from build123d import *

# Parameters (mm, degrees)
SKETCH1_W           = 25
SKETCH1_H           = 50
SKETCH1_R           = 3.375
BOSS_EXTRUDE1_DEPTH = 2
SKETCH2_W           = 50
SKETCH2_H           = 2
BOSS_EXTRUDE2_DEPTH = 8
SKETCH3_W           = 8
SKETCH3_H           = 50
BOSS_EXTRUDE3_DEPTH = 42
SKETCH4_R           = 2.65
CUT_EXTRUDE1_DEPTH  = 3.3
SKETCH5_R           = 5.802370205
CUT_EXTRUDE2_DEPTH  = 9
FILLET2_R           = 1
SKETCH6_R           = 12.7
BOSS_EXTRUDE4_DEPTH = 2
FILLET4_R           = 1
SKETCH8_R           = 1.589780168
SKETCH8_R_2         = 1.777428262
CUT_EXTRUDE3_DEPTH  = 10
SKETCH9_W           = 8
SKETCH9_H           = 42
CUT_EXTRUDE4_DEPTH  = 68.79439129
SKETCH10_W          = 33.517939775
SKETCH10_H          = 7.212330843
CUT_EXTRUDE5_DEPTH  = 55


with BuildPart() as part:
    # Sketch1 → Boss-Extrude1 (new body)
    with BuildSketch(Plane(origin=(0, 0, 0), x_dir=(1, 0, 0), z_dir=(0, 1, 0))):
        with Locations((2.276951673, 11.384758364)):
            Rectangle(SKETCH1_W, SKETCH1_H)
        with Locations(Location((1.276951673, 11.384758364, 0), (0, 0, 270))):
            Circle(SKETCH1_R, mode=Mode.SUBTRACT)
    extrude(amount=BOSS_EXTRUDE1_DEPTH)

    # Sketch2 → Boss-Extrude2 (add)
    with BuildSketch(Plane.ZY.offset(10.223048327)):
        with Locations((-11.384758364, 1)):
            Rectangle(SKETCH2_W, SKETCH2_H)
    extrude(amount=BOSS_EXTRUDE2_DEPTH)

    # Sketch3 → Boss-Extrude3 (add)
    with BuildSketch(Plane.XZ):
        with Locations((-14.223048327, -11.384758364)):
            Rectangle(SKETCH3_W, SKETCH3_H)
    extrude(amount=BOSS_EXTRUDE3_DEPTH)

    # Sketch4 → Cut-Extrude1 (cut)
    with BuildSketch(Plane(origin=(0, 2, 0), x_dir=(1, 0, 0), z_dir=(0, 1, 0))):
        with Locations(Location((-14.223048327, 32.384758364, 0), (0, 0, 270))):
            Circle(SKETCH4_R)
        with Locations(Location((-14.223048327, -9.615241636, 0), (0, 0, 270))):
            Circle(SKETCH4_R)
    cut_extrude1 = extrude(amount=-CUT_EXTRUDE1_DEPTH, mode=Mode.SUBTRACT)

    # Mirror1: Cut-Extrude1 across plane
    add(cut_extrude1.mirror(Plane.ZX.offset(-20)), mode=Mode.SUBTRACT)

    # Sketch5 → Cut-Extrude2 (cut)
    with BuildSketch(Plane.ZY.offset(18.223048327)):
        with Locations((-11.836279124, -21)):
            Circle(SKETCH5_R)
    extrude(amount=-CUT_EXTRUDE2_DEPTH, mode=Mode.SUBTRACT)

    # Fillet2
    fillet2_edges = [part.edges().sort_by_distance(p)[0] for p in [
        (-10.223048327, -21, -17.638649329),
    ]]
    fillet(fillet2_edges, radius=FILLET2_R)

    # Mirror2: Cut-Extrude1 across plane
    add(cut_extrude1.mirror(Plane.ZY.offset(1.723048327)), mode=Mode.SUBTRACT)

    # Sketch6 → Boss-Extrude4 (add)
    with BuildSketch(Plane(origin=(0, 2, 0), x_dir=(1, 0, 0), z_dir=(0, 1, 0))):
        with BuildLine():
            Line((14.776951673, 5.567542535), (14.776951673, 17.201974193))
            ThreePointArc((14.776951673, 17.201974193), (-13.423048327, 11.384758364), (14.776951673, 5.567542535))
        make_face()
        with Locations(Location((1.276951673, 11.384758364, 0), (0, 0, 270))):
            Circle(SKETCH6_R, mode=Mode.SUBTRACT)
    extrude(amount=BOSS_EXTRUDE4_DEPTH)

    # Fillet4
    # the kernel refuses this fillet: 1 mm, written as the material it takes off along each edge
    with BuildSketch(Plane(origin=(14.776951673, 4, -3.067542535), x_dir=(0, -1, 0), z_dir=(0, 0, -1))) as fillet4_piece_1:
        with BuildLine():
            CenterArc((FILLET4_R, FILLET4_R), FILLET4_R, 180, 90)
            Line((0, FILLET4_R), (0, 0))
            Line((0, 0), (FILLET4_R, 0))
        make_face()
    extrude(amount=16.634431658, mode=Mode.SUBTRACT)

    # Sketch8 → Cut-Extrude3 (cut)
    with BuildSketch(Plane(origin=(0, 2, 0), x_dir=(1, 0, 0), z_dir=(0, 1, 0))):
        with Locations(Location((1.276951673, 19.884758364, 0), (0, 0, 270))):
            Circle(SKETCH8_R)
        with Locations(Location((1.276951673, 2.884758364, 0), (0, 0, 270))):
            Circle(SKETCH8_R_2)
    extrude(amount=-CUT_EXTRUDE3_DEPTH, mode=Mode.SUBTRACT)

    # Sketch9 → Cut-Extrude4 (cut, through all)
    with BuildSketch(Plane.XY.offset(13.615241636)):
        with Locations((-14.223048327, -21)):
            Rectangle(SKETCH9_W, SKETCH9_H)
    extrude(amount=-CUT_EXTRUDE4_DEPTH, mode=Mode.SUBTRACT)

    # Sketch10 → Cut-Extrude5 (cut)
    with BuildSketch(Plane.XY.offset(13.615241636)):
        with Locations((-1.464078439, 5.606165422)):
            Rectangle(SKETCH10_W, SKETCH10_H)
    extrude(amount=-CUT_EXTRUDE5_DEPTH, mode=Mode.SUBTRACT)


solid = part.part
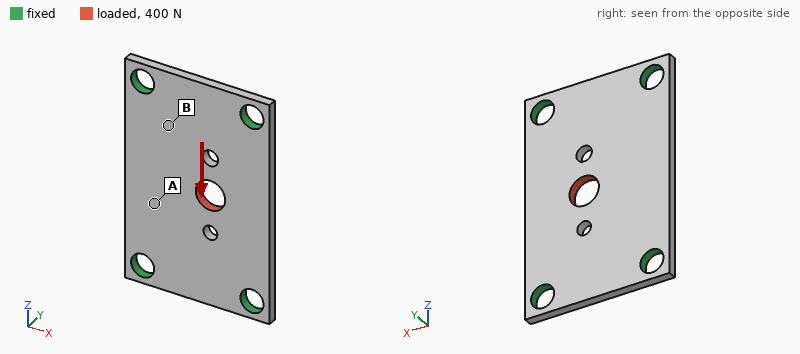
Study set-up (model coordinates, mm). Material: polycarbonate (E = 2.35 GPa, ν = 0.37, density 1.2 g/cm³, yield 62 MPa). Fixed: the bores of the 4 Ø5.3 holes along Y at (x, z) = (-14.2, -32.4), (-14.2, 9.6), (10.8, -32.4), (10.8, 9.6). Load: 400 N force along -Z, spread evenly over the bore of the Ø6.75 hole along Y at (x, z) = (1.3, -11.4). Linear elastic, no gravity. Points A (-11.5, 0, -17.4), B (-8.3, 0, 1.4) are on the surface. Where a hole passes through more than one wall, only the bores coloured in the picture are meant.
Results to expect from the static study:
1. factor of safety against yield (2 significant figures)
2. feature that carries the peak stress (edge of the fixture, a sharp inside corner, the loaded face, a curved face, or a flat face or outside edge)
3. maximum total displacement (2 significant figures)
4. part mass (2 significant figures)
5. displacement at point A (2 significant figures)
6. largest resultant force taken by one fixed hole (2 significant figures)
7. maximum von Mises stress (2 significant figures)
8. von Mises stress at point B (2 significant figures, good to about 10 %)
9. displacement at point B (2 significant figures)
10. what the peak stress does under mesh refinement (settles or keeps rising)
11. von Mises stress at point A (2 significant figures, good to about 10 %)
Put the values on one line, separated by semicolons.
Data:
3.0; a curved face; 61 µm; 3.6 g; 16 µm; 120 N; 20 MPa; 4.5 MPa; 17 µm; settles; 1.9 MPa
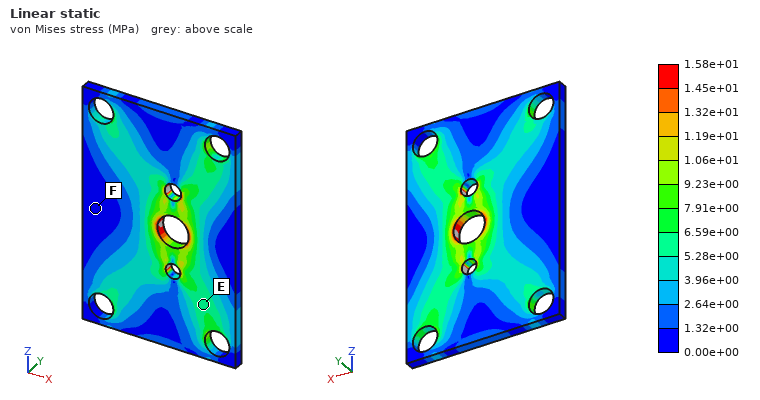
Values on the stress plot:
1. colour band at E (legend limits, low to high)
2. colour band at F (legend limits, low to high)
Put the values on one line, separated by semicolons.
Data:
5.28e+00 to 6.59e+00 MPa; 0.00e+00 to 1.32e+00 MPa
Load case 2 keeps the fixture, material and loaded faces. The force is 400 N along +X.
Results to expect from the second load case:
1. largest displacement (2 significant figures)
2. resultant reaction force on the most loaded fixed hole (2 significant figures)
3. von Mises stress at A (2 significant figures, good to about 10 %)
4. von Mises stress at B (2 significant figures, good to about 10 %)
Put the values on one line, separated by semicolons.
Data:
0.11 mm; 130 N; 4.8 MPa; 7.0 MPa
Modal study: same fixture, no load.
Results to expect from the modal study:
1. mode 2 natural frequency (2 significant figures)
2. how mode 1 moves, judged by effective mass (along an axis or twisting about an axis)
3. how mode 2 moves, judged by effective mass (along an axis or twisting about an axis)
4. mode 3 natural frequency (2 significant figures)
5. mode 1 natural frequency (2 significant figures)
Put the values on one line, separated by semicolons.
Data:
2500 Hz; along Y; twisting about Z; 3900 Hz; 1800 Hz
